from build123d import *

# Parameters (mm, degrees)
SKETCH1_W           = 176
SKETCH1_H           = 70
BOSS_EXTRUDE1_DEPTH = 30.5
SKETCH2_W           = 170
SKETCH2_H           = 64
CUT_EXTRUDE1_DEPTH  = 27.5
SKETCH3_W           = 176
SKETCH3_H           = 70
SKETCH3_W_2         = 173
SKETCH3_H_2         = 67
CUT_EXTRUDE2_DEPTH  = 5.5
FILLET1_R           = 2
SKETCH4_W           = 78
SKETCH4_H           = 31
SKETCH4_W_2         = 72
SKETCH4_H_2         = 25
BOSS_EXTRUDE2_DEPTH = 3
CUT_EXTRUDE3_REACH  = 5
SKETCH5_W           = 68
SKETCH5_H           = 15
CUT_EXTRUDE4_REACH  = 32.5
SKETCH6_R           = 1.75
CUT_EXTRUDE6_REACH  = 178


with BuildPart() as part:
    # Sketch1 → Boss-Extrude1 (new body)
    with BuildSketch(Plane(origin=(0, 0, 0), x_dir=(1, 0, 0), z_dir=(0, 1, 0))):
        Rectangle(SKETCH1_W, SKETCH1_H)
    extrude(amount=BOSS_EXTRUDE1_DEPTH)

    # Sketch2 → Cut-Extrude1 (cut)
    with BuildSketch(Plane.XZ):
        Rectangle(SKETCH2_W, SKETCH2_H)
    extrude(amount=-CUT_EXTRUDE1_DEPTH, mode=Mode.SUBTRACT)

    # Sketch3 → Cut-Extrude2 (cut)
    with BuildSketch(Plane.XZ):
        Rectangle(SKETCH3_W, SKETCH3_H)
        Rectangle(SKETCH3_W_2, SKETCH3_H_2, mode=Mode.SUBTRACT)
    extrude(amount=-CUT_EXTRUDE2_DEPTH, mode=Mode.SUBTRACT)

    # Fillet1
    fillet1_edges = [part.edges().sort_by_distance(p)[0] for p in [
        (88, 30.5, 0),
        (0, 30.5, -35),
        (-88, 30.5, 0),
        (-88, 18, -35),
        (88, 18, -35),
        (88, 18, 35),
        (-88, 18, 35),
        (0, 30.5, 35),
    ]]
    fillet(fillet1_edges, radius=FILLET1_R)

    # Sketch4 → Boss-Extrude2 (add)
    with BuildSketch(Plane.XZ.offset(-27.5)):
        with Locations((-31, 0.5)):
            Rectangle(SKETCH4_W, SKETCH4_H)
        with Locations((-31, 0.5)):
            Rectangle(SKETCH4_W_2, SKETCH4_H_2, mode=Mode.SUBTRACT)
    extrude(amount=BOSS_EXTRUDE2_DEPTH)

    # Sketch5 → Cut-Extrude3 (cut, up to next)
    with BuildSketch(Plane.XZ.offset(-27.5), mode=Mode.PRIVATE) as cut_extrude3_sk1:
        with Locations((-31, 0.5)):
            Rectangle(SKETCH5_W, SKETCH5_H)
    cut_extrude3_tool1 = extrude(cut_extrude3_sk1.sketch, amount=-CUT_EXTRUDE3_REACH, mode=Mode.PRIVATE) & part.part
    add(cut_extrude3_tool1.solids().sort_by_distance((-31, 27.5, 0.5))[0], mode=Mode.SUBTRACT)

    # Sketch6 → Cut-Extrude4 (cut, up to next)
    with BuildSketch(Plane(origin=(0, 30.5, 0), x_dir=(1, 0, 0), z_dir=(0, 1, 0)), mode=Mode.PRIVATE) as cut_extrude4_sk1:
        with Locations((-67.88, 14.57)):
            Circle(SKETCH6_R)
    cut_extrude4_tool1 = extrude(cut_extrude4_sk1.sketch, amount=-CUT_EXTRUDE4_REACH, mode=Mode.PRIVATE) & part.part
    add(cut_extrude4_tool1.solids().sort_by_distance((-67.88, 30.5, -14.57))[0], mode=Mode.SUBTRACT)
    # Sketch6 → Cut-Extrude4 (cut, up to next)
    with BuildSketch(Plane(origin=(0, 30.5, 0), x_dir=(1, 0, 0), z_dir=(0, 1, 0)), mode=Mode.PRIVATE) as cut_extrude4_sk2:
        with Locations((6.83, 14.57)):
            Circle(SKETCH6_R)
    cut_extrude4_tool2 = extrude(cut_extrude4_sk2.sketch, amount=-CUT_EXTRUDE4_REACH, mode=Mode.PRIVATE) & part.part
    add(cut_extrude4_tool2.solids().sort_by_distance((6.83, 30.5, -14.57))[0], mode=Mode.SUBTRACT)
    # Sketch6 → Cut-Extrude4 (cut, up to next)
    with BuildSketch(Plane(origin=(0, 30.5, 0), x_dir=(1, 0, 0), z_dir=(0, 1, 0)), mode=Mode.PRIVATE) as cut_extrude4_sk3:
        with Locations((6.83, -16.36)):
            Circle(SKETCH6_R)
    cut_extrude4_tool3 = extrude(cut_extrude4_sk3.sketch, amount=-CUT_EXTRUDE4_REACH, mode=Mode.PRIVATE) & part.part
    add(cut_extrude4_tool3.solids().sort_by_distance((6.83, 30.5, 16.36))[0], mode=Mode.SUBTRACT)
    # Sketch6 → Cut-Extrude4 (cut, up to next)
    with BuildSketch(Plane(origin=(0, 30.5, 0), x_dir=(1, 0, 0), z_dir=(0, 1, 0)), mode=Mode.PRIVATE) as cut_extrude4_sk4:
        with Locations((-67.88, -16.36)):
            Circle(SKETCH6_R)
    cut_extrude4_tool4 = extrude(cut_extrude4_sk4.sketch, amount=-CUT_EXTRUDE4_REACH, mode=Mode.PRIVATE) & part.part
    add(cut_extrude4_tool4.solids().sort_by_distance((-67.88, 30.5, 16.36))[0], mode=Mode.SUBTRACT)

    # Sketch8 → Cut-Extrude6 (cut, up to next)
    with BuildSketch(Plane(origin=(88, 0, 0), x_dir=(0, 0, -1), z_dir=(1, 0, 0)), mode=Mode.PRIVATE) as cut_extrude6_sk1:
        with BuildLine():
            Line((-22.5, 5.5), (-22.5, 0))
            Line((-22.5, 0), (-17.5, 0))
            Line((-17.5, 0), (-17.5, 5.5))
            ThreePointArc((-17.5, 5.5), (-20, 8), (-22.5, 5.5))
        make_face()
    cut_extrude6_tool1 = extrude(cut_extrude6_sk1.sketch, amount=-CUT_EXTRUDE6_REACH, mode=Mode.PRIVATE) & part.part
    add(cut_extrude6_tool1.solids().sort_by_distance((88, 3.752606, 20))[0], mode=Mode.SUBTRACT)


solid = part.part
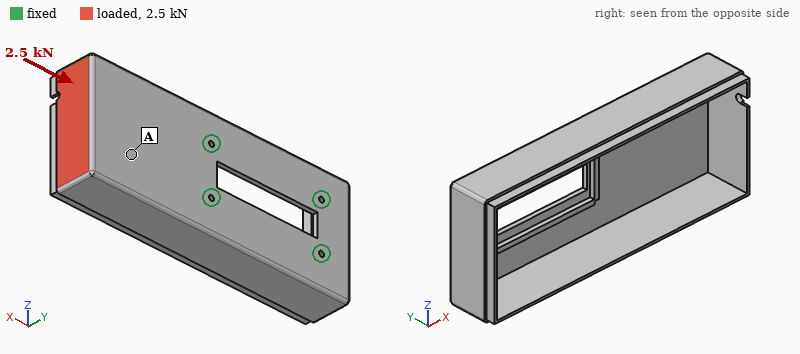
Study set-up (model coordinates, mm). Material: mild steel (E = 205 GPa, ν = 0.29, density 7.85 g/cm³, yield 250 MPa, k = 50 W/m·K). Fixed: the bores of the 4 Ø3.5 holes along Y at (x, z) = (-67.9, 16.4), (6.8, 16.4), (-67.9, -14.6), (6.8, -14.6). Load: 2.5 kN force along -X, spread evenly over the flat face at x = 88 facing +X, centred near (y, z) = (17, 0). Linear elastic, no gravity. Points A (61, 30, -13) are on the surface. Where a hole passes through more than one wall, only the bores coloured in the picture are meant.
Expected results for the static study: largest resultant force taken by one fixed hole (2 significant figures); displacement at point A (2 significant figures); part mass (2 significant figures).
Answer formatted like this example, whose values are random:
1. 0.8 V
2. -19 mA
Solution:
1. 850 N
2. 0.027 mm
3. 550 g
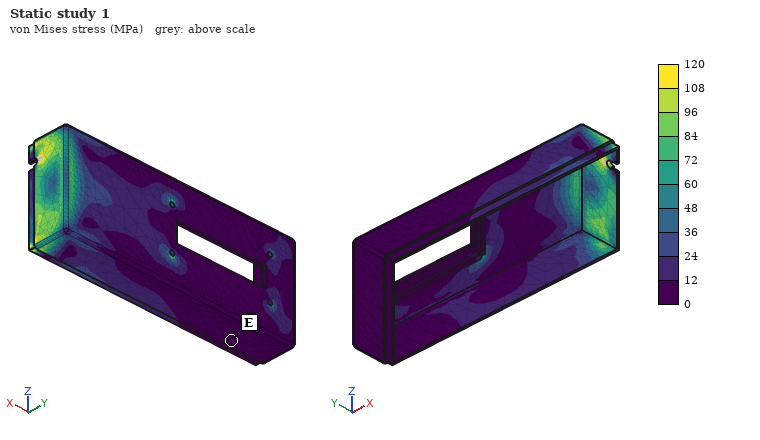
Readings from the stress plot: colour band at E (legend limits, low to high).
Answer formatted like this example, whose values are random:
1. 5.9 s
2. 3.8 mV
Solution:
1. 0 to 12 MPa
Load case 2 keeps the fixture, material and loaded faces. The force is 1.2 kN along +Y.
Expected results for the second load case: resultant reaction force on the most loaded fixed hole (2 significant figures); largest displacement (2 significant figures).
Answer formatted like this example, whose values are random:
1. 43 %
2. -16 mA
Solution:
1. 1.4 kN
2. 0.33 mm
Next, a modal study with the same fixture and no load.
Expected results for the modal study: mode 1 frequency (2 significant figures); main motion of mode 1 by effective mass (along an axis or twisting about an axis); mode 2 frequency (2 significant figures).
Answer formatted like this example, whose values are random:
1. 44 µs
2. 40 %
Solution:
1. 830 Hz
2. along Y
3. 910 Hz
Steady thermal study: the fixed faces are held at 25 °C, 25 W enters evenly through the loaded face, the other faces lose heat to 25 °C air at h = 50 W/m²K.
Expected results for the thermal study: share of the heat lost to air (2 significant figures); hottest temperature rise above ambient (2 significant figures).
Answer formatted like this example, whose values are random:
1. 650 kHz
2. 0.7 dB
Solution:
1. 89 %
2. 56 K
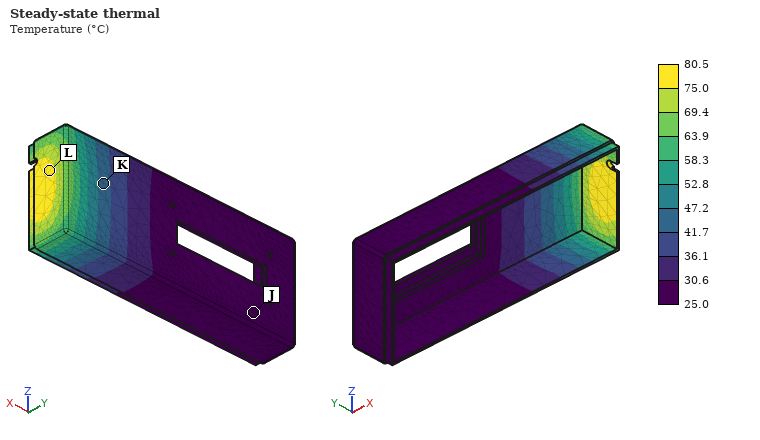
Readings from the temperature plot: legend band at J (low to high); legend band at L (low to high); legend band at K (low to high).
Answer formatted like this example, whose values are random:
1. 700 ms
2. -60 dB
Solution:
1. 25.0 to 30.6 °C
2. 75.0 to 80.5 °C
3. 41.7 to 47.2 °C
